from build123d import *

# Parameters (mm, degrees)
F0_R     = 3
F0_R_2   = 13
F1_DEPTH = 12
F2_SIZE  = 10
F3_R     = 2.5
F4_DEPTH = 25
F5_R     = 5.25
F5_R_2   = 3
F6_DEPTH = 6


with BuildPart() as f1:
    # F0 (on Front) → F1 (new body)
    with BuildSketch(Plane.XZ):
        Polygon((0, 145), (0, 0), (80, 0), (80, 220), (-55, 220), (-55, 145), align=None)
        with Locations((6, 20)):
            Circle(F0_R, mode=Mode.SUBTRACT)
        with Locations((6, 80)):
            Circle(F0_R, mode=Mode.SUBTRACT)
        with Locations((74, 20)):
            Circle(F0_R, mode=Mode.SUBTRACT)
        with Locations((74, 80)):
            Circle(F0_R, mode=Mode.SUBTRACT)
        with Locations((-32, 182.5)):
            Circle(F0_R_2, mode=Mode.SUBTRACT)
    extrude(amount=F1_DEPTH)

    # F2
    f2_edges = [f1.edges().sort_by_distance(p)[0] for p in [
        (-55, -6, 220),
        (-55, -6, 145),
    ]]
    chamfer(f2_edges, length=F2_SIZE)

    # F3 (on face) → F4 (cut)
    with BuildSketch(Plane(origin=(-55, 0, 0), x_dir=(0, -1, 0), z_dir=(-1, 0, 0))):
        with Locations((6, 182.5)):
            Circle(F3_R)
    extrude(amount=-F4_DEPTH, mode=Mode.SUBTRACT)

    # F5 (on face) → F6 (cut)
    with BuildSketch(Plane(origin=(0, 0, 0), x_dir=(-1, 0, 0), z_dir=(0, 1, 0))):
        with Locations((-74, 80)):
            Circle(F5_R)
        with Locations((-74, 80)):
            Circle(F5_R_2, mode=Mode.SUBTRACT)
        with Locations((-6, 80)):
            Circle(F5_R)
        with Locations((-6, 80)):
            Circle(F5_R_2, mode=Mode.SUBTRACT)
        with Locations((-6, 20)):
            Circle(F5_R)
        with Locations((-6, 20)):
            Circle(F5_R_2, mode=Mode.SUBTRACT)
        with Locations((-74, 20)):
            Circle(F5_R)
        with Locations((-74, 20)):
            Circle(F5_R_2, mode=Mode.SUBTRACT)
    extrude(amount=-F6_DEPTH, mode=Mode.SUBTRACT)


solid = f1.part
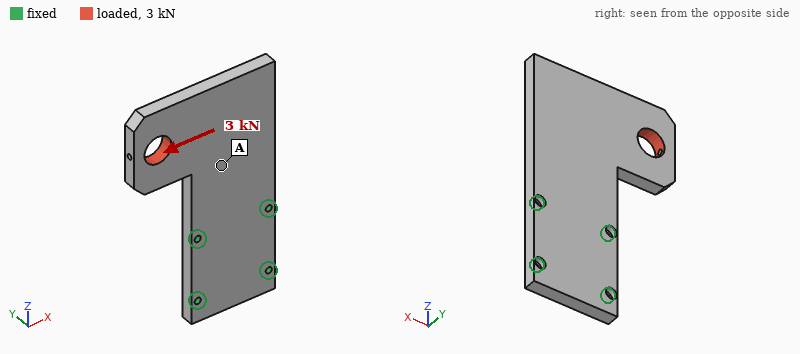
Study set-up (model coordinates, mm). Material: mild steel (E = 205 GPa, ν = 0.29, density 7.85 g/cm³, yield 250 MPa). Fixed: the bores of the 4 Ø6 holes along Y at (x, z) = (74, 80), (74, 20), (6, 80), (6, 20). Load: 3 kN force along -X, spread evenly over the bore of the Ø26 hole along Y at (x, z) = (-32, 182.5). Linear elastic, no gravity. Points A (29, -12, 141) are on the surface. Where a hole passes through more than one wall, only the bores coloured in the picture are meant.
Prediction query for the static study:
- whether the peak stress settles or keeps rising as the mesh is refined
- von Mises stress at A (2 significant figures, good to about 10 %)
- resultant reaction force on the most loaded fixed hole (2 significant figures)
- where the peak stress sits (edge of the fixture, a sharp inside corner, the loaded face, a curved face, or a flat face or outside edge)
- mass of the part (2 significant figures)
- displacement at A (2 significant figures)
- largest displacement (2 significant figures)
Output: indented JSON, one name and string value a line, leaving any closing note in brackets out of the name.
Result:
{
  "whether the peak stress settles or keeps rising as the mesh is refined": "keeps rising",
  "von Mises stress at A": "8.7 MPa",
  "resultant reaction force on the most loaded fixed hole": "4.2 kN",
  "where the peak stress sits": "edge of the fixture",
  "mass of the part": "2.0 kg",
  "displacement at A": "9.9 µm",
  "largest displacement": "32 µm"
}
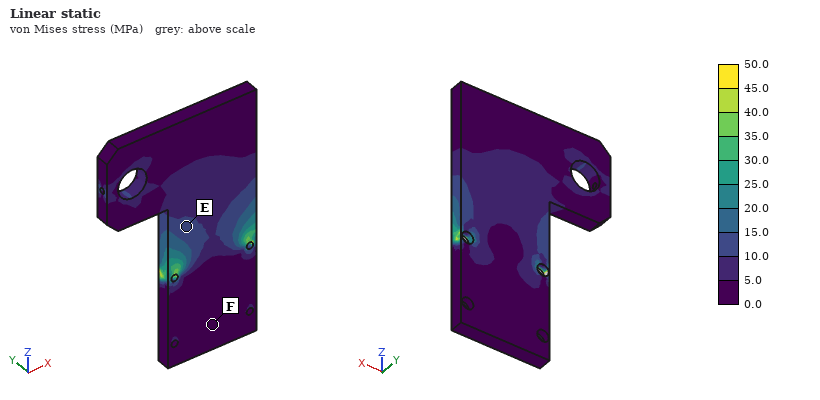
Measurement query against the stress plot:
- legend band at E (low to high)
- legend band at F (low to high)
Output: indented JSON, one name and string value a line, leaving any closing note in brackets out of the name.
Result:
{
  "legend band at E": "10.0 to 15.0 MPa",
  "legend band at F": "0.0 to 5.0 MPa"
}
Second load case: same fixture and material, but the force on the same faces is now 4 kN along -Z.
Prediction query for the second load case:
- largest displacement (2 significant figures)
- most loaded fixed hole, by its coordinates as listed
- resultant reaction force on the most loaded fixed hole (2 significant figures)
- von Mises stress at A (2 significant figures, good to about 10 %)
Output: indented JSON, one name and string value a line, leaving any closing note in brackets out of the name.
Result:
{
  "largest displacement": "48 µm",
  "most loaded fixed hole, by its coordinates as listed": "(6, 80)",
  "resultant reaction force on the most loaded fixed hole": "5.0 kN",
  "von Mises stress at A": "6.9 MPa"
}
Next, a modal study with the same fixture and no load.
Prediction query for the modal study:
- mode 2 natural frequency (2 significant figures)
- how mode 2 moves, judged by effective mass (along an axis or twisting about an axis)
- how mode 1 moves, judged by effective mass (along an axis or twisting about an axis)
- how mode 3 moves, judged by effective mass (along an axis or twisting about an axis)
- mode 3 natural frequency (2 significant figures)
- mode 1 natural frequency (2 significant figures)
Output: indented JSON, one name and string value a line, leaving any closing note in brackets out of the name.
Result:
{
  "mode 2 natural frequency": "890 Hz",
  "how mode 2 moves, judged by effective mass": "twisting about Z",
  "how mode 1 moves, judged by effective mass": "along Y",
  "how mode 3 moves, judged by effective mass": "along X",
  "mode 3 natural frequency": "1900 Hz",
  "mode 1 natural frequency": "330 Hz"
}
